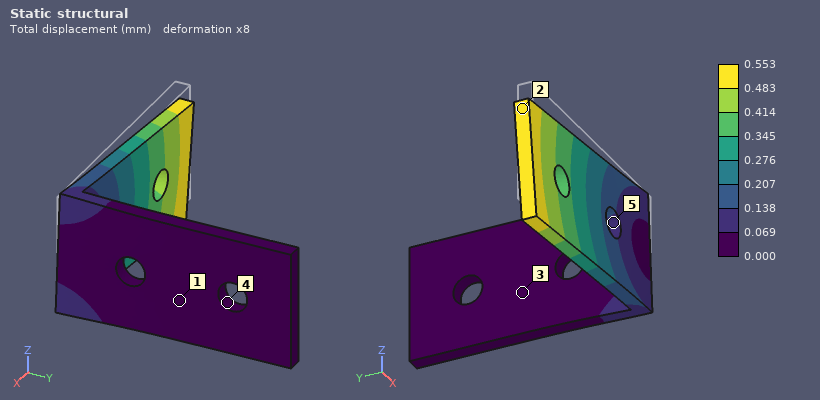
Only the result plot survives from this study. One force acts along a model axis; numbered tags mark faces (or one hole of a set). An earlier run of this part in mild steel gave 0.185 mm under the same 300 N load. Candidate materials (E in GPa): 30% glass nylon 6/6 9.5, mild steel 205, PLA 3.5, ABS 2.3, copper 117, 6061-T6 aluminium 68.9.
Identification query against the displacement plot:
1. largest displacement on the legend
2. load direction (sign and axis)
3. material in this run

0.553 mm
-Z
6061-T6 aluminium
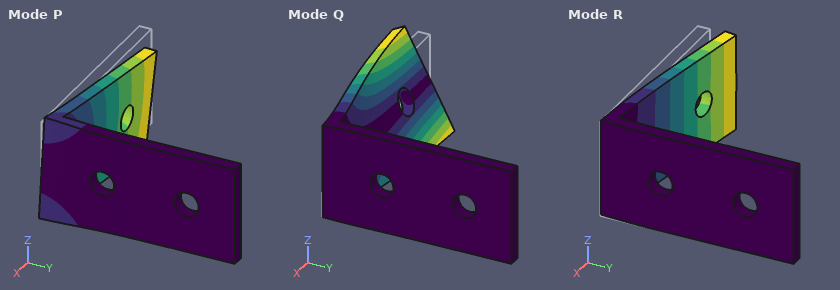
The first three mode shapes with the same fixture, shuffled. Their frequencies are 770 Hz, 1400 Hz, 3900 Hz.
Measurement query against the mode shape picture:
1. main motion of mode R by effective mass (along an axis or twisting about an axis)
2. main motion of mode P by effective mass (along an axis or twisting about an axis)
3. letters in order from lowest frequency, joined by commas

along Y
along Z
R, P, Q
